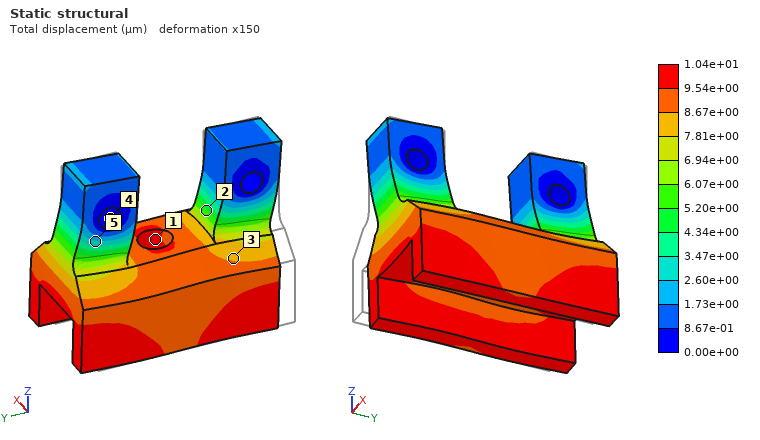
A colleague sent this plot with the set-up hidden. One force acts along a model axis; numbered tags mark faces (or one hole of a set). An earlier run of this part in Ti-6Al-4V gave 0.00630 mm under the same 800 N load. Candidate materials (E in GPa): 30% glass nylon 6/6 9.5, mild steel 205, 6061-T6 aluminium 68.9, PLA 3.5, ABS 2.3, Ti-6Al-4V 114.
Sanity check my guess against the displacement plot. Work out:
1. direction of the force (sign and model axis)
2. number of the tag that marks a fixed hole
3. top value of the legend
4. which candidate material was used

+Y
4
1.04e+01 µm
6061-T6 aluminium
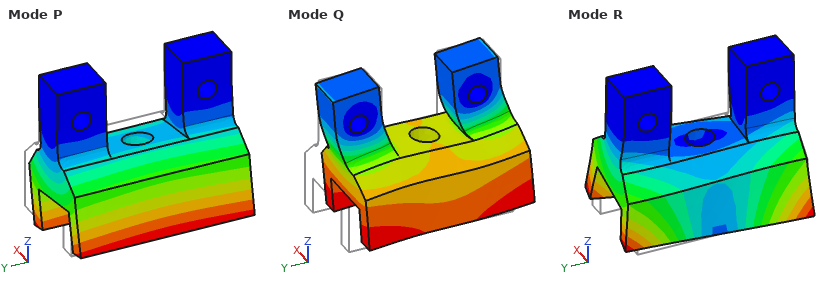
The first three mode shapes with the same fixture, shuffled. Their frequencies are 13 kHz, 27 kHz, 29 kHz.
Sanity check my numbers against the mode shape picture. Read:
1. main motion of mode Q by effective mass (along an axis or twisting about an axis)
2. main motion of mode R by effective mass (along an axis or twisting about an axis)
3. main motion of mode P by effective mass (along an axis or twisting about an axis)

along Y
twisting about Z
along X
